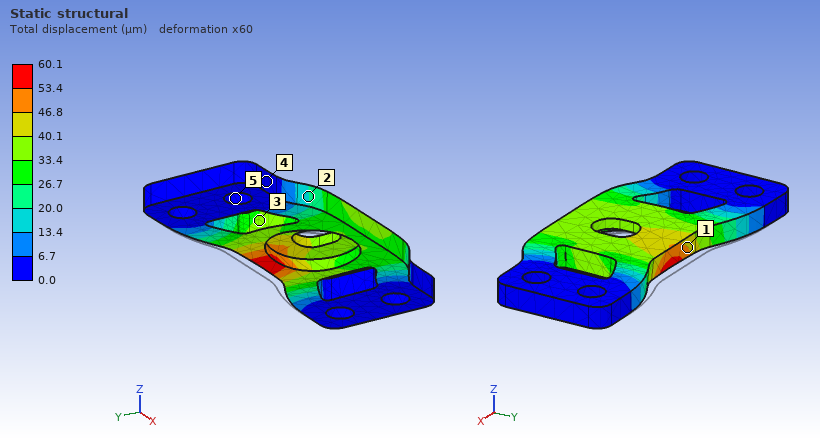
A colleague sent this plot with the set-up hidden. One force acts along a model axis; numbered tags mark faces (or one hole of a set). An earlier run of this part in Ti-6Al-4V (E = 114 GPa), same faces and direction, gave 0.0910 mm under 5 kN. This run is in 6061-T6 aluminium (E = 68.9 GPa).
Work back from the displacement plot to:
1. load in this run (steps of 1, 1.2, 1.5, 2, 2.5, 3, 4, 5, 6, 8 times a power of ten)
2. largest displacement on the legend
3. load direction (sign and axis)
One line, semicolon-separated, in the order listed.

2 kN; 60.1 µm; -Y
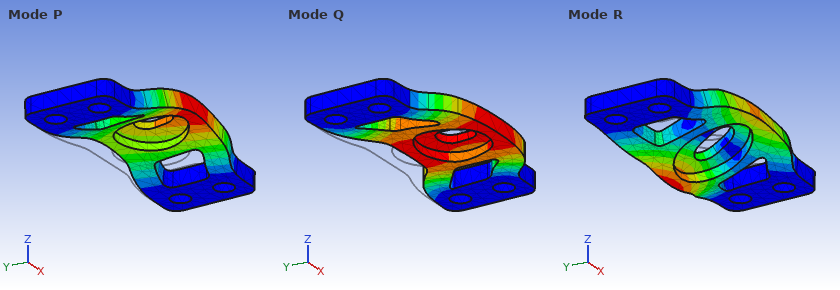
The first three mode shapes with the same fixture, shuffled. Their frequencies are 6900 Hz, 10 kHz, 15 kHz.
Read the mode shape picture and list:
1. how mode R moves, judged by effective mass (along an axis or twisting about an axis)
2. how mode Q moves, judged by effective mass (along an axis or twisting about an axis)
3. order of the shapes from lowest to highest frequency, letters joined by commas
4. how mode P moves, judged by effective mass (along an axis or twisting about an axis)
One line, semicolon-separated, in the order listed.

twisting about X; along Y; P, R, Q; along Z
